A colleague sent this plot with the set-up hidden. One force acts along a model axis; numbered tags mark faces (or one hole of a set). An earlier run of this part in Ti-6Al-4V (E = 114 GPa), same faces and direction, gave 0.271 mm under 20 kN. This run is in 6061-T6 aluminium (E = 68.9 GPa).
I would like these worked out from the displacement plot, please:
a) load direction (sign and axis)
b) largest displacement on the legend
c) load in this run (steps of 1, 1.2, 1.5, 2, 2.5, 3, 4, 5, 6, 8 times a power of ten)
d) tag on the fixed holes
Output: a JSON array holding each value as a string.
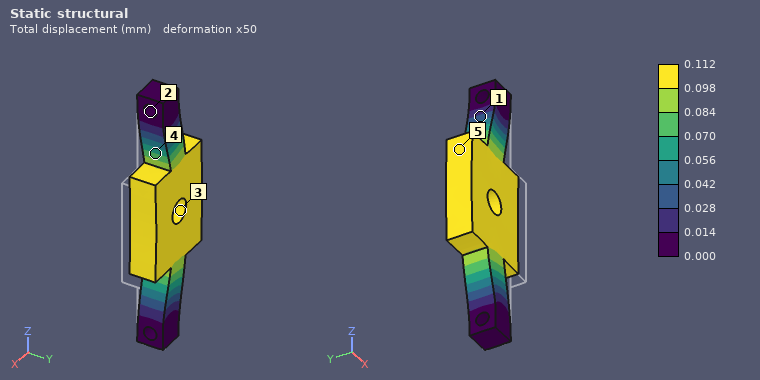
["-X", "0.112 mm", "5 kN", "2"]
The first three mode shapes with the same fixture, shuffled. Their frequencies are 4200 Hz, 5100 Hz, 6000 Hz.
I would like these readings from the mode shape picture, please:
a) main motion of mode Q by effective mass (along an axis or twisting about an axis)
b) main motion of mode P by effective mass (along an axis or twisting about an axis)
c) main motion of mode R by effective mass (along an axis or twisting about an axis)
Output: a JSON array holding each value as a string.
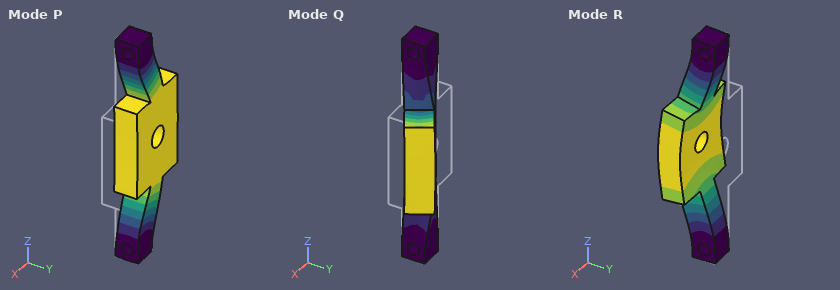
["twisting about Z", "along X", "along Y"]
